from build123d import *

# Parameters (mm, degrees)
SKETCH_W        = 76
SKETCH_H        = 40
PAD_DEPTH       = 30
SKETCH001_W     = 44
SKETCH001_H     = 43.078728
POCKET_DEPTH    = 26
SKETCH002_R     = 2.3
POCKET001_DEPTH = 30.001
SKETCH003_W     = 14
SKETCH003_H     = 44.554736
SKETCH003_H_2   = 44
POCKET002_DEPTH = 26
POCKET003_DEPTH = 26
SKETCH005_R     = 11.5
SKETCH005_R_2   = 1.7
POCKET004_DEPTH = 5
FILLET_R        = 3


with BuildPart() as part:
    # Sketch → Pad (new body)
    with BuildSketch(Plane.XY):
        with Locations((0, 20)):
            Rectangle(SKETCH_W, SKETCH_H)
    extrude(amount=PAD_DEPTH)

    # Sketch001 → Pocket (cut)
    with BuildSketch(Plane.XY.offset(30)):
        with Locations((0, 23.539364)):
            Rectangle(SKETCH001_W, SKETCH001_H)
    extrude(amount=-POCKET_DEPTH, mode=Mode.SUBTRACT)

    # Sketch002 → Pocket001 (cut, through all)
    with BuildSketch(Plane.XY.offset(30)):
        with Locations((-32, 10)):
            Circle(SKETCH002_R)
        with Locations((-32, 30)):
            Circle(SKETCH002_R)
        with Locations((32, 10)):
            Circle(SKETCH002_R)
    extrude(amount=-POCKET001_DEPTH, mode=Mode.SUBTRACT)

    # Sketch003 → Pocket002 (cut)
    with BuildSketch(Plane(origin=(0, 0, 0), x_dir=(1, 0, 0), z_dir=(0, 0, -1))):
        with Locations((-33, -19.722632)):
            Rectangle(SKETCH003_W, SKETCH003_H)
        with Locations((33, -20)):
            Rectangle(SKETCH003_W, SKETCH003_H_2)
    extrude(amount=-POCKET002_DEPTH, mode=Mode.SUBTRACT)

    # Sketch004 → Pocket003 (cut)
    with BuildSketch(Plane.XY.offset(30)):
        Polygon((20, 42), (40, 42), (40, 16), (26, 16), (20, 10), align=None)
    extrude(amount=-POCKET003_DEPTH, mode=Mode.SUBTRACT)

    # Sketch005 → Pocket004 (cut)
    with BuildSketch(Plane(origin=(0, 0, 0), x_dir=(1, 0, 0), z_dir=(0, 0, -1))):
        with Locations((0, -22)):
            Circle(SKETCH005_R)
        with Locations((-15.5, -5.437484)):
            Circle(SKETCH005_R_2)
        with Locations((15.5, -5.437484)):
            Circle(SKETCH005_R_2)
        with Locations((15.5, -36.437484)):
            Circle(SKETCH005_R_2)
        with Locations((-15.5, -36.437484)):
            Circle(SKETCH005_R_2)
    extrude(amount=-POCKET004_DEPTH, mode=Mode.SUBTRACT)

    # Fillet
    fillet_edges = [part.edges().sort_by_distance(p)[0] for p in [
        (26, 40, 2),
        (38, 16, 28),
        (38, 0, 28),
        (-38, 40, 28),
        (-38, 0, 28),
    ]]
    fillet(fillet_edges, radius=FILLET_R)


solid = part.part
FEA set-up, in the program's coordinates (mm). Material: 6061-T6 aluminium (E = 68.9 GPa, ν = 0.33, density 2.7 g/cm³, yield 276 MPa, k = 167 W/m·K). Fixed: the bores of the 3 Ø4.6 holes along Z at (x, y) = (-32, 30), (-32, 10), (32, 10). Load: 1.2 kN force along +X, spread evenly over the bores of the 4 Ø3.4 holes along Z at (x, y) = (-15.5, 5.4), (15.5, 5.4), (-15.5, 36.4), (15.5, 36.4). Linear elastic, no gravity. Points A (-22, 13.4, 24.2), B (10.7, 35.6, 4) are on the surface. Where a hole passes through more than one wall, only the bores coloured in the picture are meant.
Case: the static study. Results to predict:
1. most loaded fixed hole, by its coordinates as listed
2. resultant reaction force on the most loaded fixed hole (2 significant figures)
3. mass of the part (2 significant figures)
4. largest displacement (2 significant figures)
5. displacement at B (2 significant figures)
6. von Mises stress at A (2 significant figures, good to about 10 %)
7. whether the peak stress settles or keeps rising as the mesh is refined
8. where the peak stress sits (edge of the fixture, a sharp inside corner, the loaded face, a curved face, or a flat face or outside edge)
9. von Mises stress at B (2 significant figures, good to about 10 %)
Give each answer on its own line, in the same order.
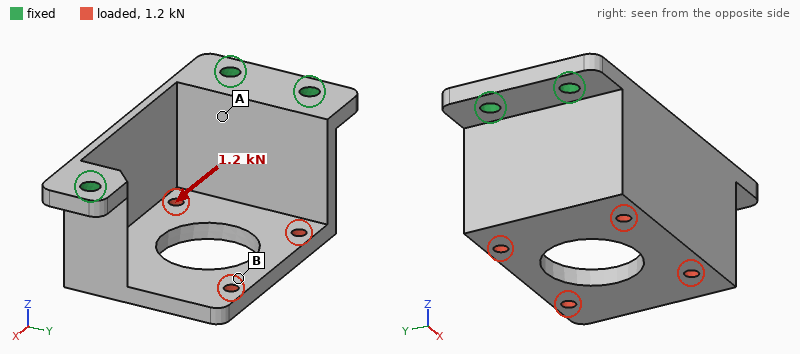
(-32, 10)
890 N
46 g
0.22 mm
0.18 mm
35 MPa
keeps rising
edge of the fixture
10.0 MPa
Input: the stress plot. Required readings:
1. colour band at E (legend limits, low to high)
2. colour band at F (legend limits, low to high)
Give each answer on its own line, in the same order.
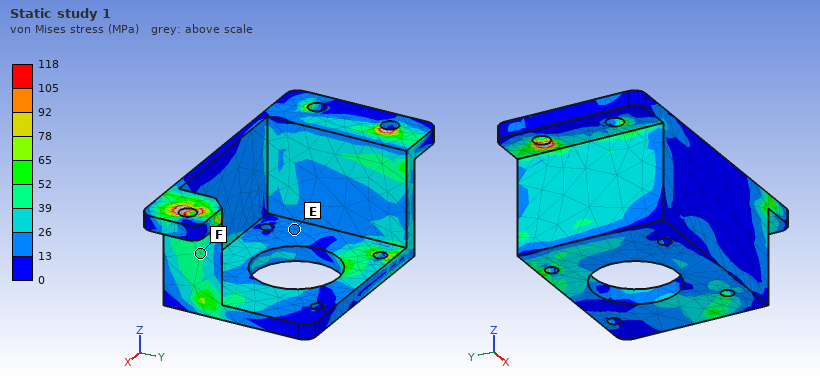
13 to 26 MPa
39 to 52 MPa
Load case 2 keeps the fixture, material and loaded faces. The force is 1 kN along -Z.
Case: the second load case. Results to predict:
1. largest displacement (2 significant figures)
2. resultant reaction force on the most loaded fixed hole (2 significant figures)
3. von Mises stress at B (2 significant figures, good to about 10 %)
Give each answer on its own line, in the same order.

0.24 mm
560 N
53 MPa
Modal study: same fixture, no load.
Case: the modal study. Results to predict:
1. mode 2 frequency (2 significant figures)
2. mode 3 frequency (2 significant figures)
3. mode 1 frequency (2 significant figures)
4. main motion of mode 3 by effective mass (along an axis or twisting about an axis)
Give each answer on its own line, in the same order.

3600 Hz
4900 Hz
2700 Hz
along Y
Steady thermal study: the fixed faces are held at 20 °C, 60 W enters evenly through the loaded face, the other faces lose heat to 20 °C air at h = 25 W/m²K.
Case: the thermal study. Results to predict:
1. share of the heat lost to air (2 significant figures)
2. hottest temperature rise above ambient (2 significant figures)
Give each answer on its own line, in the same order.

15 %
78 K
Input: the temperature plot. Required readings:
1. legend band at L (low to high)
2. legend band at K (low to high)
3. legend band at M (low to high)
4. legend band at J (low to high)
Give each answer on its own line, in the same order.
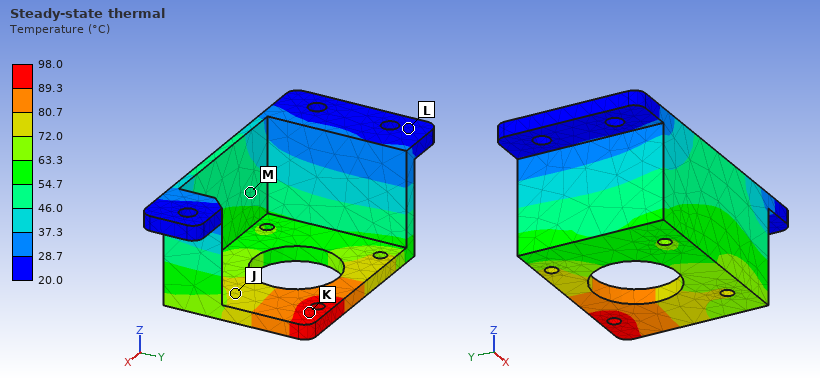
20.0 to 28.7 °C
89.3 to 98.0 °C
46.0 to 54.7 °C
72.0 to 80.7 °C
